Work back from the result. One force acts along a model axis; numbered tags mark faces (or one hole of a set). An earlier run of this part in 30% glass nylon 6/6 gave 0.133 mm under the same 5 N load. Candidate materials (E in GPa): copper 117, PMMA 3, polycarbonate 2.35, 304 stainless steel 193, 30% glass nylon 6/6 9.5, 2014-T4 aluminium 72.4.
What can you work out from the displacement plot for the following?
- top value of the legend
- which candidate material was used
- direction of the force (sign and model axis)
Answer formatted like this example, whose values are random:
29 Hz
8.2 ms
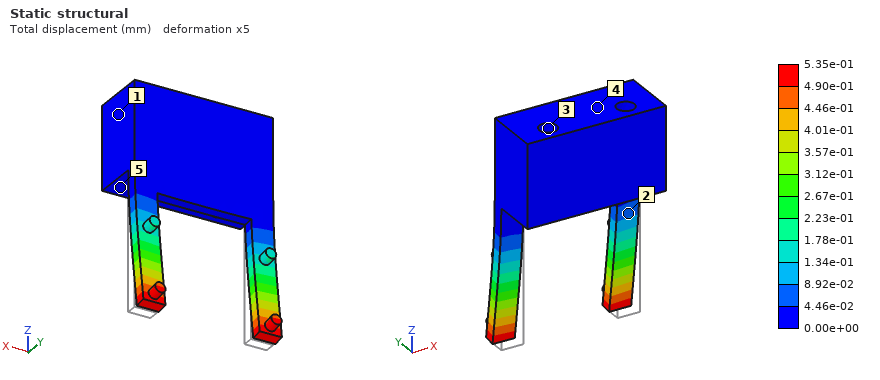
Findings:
5.35e-01 mm
polycarbonate
+Y
